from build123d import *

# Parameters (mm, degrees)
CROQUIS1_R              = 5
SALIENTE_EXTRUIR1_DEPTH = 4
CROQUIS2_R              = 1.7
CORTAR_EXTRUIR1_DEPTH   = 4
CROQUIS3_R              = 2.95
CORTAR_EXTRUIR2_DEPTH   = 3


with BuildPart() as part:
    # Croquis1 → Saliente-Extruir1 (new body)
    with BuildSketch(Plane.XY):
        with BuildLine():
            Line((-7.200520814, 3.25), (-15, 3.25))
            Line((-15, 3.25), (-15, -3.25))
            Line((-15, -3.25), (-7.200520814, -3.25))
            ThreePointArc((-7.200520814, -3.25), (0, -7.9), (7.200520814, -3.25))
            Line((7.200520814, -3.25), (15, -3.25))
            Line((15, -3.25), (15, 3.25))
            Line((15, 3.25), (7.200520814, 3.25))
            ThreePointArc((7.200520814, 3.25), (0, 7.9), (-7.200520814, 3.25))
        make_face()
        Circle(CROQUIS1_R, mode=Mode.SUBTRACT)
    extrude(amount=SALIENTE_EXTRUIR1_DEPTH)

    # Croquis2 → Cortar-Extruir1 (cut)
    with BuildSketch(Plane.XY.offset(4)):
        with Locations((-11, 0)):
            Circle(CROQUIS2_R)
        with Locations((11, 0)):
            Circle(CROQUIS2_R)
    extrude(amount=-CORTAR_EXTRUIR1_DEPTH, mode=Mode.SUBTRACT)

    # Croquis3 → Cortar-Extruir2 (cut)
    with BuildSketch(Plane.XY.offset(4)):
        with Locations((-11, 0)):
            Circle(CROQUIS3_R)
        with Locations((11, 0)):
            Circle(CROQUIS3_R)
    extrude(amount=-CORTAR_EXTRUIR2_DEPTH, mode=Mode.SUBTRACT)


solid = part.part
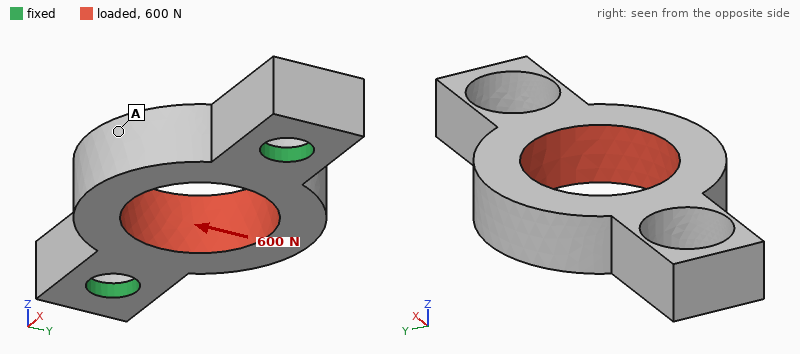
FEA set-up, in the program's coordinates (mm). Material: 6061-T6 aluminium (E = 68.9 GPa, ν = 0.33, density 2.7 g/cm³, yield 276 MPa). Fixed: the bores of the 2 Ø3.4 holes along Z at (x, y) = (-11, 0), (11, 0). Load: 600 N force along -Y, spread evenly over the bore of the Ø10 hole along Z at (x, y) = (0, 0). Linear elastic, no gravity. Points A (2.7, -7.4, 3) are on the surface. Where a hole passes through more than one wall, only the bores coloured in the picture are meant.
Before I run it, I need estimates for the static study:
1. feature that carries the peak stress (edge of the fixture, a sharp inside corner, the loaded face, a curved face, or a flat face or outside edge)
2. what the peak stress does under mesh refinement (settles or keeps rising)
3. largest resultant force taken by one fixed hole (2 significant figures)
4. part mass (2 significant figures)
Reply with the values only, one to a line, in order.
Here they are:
edge of the fixture
keeps rising
300 N
1.8 g
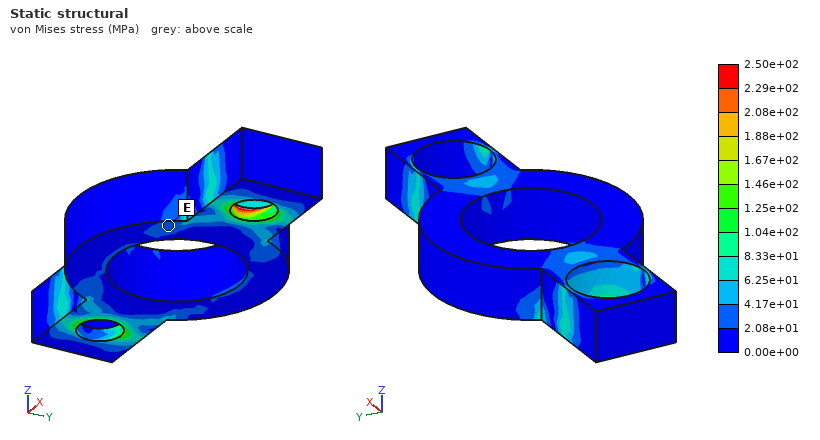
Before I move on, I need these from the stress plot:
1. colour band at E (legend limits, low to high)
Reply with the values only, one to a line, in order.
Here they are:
2.08e+01 to 4.17e+01 MPa
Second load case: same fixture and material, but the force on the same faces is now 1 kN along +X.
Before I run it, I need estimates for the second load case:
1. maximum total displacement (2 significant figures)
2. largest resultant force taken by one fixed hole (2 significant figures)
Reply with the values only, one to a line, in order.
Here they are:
8.0 µm
500 N
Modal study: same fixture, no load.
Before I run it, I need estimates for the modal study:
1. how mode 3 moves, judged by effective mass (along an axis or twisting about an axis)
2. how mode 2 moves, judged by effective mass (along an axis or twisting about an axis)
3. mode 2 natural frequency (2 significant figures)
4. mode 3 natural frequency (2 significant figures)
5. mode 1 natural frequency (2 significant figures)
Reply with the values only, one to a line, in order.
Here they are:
along Y
along Z
20 kHz
43 kHz
14 kHz
